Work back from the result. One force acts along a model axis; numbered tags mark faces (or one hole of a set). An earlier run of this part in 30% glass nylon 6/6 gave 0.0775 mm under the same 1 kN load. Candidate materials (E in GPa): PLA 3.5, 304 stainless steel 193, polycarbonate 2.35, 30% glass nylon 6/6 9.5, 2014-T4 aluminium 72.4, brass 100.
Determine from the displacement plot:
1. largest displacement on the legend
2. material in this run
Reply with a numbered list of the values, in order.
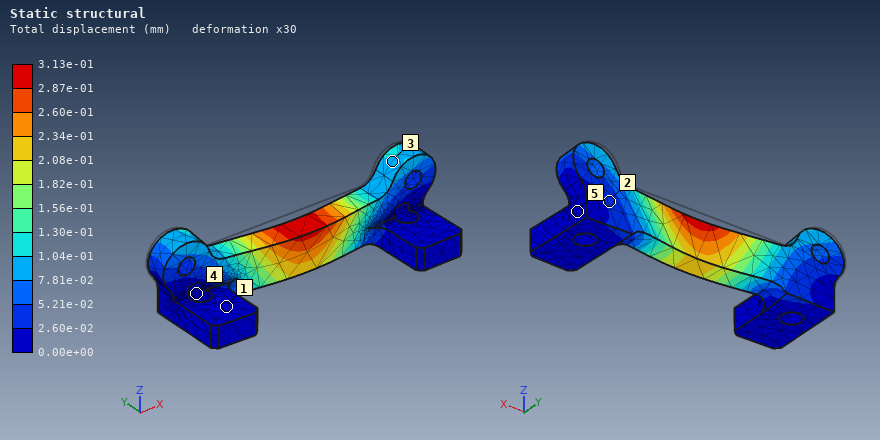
1. 3.13e-01 mm
2. polycarbonate
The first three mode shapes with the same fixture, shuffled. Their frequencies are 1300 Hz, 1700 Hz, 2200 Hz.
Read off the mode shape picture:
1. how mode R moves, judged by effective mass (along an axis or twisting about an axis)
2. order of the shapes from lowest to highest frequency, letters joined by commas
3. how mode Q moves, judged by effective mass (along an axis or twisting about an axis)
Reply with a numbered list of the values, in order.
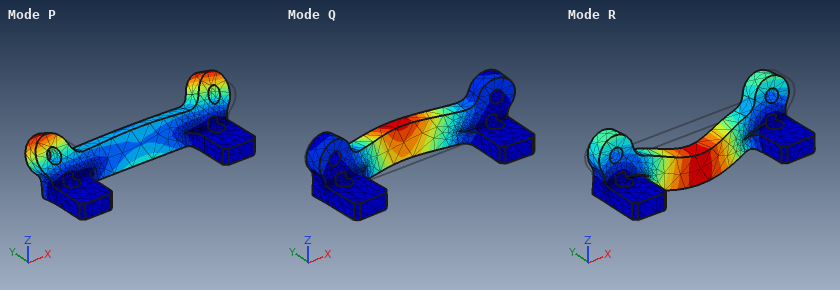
1. along Z
2. Q, R, P
3. along Y
